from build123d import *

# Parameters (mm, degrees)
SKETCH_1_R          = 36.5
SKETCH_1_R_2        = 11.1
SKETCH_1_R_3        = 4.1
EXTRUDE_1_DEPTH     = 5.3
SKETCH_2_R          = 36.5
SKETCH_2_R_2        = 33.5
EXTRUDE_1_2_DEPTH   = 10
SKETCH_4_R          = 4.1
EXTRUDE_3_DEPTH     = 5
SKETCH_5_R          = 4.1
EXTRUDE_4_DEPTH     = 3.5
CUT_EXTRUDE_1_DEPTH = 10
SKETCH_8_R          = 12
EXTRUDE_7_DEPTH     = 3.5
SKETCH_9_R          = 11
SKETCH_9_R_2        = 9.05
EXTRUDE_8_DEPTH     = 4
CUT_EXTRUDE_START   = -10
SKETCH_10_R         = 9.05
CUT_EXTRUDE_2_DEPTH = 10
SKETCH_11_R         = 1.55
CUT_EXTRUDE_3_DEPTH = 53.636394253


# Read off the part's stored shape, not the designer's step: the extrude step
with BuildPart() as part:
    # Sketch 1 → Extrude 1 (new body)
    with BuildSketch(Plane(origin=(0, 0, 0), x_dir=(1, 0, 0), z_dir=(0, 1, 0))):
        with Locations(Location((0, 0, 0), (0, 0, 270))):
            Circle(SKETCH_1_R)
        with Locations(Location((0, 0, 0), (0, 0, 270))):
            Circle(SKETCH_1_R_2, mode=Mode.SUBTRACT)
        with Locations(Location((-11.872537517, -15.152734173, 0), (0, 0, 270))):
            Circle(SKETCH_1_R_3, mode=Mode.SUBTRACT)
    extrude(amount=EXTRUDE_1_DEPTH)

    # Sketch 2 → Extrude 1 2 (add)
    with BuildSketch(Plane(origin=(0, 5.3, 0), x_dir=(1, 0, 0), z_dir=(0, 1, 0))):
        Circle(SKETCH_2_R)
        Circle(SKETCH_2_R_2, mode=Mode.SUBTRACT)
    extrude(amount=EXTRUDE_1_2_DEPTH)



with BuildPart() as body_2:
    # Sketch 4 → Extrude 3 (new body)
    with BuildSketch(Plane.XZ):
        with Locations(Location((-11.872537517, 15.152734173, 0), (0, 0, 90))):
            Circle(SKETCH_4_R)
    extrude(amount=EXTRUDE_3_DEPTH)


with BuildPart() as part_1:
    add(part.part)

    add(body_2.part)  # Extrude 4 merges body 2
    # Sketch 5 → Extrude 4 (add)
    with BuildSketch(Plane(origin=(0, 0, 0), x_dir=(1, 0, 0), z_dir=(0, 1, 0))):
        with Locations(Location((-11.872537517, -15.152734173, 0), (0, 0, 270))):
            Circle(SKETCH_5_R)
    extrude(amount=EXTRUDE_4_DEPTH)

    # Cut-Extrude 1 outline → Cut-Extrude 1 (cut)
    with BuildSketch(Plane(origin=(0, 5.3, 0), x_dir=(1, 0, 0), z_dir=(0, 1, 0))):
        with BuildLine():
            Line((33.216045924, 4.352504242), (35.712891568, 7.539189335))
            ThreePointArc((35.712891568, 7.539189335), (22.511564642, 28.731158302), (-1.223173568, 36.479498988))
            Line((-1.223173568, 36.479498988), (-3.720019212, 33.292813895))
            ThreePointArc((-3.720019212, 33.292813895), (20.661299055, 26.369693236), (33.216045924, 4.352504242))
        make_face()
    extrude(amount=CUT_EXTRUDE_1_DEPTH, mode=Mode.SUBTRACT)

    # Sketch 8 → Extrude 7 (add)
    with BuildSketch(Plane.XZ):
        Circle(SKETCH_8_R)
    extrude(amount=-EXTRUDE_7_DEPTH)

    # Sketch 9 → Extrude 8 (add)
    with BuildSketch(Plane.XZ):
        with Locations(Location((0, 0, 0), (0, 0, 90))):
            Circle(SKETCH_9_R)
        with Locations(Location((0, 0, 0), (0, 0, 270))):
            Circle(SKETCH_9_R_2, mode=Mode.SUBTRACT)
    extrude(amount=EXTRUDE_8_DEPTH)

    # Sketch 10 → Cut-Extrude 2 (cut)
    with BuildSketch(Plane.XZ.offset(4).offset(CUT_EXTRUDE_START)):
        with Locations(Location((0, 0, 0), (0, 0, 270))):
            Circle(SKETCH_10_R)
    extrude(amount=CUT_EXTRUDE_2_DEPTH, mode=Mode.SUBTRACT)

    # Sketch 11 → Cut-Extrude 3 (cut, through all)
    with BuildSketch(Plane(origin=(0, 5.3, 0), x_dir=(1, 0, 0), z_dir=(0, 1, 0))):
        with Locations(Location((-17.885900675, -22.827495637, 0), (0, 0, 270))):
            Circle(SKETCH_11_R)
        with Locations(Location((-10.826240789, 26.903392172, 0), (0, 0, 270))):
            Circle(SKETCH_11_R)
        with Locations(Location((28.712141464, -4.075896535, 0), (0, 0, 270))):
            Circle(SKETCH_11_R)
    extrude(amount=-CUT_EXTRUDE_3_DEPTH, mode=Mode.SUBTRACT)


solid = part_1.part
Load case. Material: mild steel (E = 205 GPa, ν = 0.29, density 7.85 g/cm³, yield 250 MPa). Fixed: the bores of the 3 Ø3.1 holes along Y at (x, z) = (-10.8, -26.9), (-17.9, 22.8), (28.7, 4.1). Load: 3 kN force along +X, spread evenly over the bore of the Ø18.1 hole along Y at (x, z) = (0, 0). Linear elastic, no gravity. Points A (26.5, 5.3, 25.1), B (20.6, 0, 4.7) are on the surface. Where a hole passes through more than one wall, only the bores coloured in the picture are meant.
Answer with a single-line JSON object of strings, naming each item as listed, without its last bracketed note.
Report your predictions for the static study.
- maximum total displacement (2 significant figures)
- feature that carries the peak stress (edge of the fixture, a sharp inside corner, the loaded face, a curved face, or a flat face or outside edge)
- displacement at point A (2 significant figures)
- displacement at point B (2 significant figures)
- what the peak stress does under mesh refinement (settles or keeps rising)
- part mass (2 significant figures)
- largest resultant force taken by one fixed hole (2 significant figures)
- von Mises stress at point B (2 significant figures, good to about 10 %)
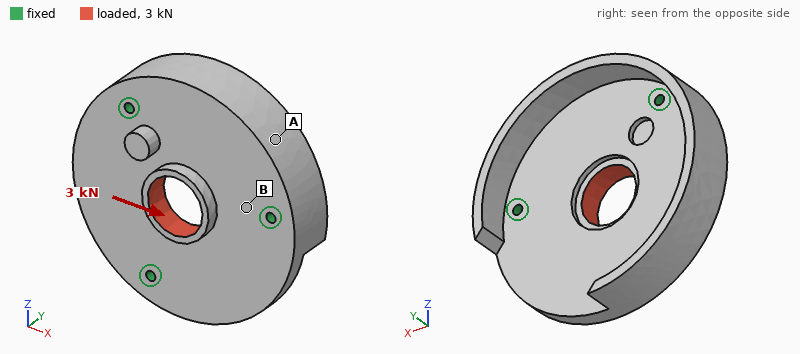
{"maximum total displacement": "4.7 µm", "feature that carries the peak stress": "edge of the fixture", "displacement at point A": "0.78 µm", "displacement at point B": "0.74 µm", "what the peak stress does under mesh refinement": "keeps rising", "part mass": "210 g", "largest resultant force taken by one fixed hole": "1.0 kN", "von Mises stress at point B": "16 MPa"}
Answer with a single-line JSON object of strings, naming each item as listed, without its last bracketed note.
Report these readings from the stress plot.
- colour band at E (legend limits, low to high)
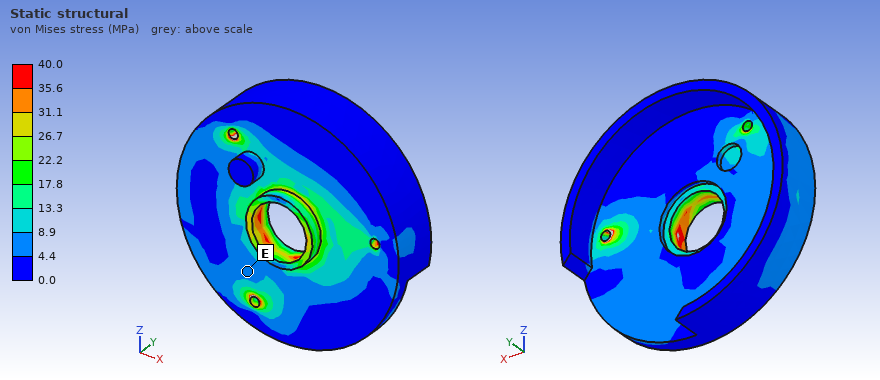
{"colour band at E": "4.4 to 8.9 MPa"}
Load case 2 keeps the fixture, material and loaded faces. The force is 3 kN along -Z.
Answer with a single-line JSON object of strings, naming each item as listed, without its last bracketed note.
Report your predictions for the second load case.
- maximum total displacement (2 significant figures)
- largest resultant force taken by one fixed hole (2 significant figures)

{"maximum total displacement": "4.6 µm", "largest resultant force taken by one fixed hole": "1.0 kN"}
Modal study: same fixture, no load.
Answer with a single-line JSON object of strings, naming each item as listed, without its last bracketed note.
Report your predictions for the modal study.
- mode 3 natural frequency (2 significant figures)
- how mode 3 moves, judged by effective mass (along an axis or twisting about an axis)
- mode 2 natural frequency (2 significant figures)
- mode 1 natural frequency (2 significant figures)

{"mode 3 natural frequency": "8300 Hz", "how mode 3 moves, judged by effective mass": "along Y", "mode 2 natural frequency": "6300 Hz", "mode 1 natural frequency": "5600 Hz"}
